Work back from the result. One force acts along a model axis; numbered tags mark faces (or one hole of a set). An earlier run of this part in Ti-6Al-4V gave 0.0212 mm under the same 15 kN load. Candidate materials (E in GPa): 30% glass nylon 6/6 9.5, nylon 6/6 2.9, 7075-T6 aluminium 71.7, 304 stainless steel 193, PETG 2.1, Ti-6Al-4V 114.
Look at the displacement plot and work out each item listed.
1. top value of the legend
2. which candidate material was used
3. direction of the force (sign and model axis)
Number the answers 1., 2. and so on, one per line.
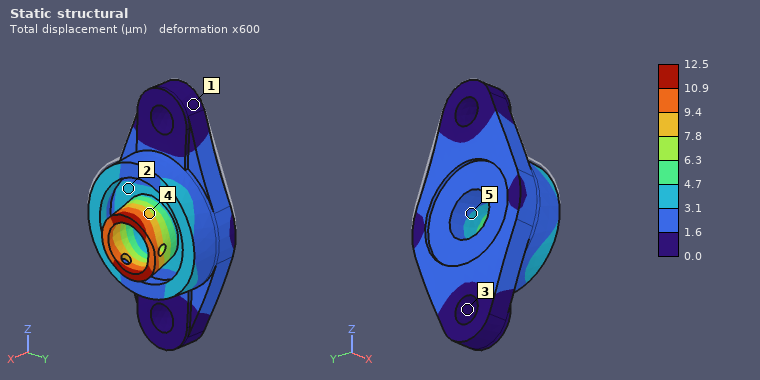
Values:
1. 12.5 µm
2. 304 stainless steel
3. -Z
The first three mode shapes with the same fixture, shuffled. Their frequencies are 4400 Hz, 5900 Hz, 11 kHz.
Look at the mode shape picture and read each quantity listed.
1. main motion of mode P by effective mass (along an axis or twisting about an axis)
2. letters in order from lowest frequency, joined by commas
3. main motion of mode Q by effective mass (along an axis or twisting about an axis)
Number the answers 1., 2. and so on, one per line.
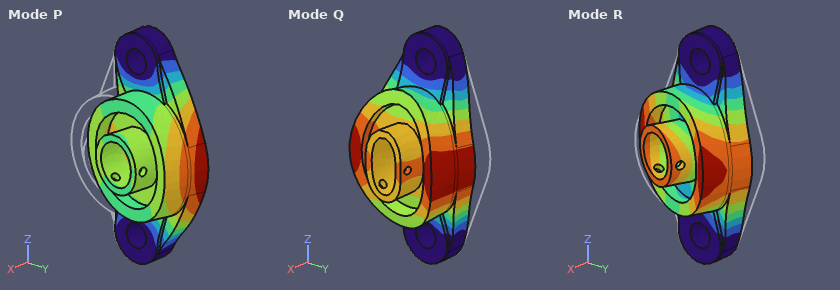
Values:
1. along Y
2. R, Q, P
3. along X
